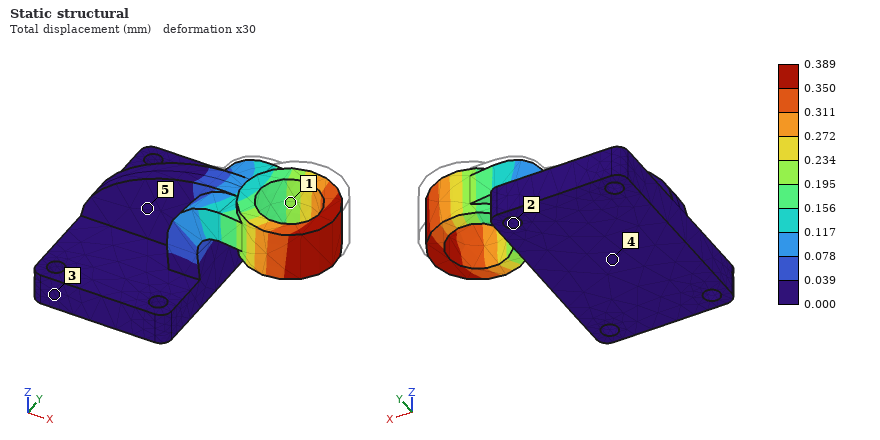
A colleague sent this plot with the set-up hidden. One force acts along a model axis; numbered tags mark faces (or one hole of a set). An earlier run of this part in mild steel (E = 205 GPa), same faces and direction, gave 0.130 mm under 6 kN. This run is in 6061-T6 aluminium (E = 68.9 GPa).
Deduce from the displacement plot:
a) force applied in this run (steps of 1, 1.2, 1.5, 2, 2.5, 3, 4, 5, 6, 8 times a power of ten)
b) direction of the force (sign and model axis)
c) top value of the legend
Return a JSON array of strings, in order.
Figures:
["6 kN", "-Y", "0.389 mm"]
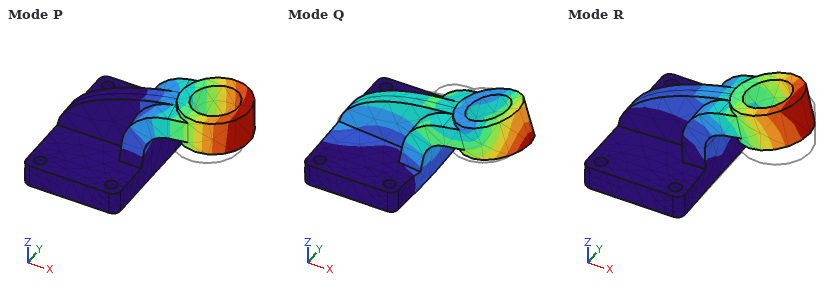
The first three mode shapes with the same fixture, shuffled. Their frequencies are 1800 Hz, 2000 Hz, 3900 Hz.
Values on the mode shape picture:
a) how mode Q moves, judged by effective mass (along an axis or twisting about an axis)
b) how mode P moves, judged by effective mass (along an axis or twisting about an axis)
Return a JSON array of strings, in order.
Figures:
["along X", "along Y"]
